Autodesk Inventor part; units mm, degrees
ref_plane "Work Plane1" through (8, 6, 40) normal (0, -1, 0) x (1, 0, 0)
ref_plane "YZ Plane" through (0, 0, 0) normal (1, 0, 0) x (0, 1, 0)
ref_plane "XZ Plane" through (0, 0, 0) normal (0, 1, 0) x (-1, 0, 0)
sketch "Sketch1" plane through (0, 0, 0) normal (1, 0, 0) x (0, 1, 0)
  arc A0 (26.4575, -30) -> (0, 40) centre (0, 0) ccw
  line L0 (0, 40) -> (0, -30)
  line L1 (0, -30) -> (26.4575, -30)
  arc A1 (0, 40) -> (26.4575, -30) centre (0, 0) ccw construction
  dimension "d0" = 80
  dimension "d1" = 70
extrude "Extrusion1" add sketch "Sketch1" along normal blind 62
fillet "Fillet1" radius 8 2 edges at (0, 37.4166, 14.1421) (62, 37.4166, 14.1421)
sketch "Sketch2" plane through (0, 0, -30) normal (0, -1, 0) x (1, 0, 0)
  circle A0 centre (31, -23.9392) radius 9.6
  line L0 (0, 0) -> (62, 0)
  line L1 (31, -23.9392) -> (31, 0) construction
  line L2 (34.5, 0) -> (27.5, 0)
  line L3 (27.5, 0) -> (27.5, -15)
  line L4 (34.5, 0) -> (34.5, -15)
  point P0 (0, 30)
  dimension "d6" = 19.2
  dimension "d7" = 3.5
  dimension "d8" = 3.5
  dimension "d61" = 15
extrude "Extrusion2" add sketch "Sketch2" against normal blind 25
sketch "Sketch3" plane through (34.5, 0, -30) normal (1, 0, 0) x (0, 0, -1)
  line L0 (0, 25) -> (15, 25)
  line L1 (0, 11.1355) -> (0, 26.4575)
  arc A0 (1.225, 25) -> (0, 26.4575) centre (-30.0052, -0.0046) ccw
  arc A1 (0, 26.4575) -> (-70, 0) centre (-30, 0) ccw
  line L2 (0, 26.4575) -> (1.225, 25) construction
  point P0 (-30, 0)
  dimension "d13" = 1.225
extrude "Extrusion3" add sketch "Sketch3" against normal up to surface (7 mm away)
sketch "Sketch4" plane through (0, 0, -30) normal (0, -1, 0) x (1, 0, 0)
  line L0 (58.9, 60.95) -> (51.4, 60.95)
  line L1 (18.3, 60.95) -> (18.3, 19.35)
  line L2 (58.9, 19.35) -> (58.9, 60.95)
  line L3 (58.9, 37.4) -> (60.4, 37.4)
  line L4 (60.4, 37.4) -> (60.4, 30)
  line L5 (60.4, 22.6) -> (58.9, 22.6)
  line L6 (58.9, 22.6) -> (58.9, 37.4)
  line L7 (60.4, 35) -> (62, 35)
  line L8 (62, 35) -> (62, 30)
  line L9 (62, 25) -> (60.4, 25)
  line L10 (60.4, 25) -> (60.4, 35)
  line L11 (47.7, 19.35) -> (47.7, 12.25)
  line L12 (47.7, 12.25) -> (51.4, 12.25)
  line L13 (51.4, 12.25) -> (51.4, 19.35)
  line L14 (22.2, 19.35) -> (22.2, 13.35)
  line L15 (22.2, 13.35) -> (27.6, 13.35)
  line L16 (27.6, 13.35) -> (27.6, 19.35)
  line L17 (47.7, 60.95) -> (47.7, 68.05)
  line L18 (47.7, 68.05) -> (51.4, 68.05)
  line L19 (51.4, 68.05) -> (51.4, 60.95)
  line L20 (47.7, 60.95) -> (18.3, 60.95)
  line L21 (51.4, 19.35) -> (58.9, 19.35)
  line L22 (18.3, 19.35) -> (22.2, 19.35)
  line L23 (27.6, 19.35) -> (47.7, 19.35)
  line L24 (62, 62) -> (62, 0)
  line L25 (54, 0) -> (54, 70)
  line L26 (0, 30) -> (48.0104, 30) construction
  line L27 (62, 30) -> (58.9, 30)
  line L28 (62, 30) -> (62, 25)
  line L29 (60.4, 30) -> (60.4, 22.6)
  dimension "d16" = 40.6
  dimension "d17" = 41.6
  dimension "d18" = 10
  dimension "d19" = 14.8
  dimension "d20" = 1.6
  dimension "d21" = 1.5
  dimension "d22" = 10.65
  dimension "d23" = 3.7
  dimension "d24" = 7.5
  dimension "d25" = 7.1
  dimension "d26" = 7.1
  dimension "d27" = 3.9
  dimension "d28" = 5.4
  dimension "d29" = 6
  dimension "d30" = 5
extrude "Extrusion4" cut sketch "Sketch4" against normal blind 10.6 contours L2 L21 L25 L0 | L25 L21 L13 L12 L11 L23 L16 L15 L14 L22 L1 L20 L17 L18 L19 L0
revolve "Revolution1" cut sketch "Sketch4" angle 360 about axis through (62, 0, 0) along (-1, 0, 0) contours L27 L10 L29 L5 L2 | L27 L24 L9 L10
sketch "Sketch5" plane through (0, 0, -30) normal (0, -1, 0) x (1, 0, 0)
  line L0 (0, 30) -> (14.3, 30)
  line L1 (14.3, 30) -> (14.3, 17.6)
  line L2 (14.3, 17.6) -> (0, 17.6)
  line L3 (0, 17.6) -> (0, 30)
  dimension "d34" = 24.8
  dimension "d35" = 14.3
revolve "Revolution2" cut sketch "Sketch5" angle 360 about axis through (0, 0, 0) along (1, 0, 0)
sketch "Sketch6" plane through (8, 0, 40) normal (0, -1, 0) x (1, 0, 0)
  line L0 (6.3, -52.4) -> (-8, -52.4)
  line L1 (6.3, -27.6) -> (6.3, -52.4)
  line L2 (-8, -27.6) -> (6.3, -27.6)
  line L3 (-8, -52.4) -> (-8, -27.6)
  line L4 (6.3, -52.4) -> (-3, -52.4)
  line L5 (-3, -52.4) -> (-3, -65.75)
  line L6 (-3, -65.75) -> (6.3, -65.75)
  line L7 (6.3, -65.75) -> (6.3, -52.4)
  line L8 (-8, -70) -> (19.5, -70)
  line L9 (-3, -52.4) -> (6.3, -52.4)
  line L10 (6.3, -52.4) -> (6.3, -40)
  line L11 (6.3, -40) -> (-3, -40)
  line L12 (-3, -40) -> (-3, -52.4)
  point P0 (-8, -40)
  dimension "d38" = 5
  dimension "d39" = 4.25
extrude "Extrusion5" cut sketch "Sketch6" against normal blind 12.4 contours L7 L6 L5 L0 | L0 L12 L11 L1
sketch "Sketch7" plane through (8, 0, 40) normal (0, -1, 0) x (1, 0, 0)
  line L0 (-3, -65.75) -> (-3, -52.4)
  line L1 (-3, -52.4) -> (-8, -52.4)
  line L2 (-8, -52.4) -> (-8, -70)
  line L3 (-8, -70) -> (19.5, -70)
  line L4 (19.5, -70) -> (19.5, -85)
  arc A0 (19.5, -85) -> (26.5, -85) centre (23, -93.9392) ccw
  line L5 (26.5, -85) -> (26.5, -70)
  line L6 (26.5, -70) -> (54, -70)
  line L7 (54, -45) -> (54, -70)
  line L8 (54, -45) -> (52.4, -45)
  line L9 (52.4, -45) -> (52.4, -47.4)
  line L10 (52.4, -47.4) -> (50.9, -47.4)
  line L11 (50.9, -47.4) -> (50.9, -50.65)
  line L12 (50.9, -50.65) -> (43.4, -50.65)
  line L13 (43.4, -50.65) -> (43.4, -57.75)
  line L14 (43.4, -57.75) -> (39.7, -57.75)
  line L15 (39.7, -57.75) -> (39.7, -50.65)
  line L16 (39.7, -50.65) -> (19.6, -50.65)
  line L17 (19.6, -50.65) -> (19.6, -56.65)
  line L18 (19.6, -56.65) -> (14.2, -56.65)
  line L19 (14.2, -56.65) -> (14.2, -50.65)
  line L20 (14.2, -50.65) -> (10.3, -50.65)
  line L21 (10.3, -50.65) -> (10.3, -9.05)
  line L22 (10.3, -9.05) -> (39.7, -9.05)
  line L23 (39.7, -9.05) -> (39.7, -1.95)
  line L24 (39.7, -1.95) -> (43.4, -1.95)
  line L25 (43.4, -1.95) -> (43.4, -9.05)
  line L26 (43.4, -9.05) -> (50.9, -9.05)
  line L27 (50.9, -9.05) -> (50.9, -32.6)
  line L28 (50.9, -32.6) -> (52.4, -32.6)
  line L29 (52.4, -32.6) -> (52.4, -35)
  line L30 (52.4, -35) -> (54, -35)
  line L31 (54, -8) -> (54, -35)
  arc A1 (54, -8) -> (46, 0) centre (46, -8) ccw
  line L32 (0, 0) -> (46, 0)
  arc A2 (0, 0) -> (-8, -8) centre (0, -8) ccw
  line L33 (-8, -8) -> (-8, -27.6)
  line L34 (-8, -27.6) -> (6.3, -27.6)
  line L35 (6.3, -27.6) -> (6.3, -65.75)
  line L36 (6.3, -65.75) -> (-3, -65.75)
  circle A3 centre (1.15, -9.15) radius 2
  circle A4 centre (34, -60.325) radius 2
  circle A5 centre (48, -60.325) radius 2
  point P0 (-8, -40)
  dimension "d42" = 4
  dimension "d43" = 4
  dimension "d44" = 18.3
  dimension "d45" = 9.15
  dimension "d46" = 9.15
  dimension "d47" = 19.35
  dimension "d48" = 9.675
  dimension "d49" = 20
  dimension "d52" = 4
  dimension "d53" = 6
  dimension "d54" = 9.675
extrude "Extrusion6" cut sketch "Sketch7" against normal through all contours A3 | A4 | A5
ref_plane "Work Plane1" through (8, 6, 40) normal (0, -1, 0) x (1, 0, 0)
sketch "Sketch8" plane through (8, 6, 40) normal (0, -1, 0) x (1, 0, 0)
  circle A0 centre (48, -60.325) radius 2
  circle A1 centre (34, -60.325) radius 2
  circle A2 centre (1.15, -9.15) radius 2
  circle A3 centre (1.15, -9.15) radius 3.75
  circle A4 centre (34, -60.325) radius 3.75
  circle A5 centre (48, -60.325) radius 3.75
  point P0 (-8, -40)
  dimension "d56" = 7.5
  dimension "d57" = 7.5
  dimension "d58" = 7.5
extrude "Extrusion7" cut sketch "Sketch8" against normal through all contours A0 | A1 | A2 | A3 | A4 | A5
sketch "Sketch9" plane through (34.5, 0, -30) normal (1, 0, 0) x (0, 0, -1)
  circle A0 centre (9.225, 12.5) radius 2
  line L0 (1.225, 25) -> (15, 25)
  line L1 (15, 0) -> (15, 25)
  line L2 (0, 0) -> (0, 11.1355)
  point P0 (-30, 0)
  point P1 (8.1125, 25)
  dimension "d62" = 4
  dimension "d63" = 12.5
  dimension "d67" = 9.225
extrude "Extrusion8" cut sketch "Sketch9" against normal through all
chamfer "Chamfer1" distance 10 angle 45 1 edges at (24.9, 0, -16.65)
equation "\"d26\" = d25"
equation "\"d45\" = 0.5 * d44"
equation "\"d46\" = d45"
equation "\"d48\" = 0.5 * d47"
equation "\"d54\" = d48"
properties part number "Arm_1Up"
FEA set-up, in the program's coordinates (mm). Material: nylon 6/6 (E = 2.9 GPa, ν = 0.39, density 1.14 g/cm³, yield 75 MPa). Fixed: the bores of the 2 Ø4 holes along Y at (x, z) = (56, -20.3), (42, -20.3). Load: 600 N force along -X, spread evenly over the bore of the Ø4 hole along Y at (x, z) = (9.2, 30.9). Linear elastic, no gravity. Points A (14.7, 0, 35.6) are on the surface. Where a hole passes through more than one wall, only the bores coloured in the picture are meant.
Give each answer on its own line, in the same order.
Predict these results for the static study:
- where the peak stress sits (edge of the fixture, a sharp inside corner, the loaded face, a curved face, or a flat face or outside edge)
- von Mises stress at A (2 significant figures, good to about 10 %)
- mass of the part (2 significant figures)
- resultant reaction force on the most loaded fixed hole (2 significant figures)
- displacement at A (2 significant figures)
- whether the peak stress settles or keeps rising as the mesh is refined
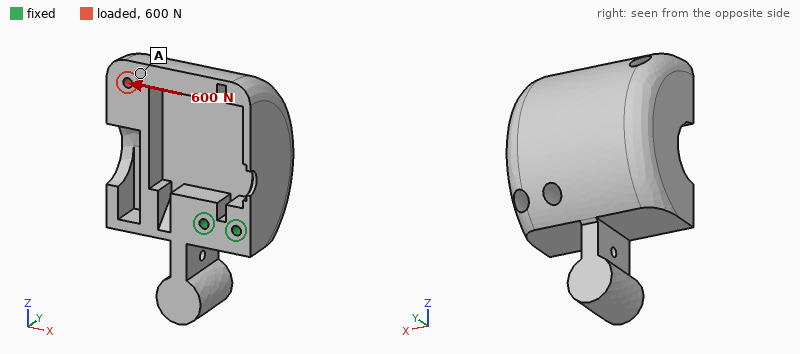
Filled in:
edge of the fixture
4.8 MPa
140 g
1.8 kN
1.2 mm
keeps rising
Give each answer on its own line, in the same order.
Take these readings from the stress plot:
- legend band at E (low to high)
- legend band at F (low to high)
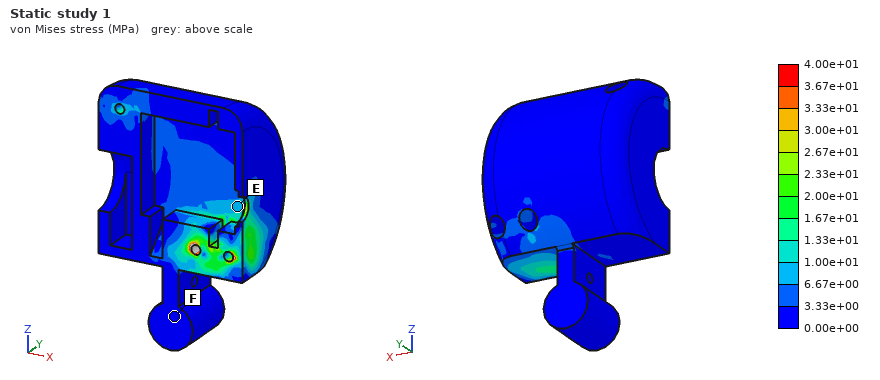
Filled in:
6.67e+00 to 1.00e+01 MPa
0.00e+00 to 3.33e+00 MPa
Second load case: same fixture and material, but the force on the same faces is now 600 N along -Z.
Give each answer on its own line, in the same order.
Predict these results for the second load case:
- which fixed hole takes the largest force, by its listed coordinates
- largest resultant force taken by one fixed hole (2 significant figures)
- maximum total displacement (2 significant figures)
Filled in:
(42, -20.3)
1.7 kN
0.94 mm
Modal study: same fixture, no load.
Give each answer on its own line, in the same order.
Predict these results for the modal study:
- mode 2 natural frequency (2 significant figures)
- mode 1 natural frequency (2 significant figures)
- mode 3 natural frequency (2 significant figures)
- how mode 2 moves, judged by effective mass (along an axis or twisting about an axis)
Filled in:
480 Hz
300 Hz
740 Hz
along X
